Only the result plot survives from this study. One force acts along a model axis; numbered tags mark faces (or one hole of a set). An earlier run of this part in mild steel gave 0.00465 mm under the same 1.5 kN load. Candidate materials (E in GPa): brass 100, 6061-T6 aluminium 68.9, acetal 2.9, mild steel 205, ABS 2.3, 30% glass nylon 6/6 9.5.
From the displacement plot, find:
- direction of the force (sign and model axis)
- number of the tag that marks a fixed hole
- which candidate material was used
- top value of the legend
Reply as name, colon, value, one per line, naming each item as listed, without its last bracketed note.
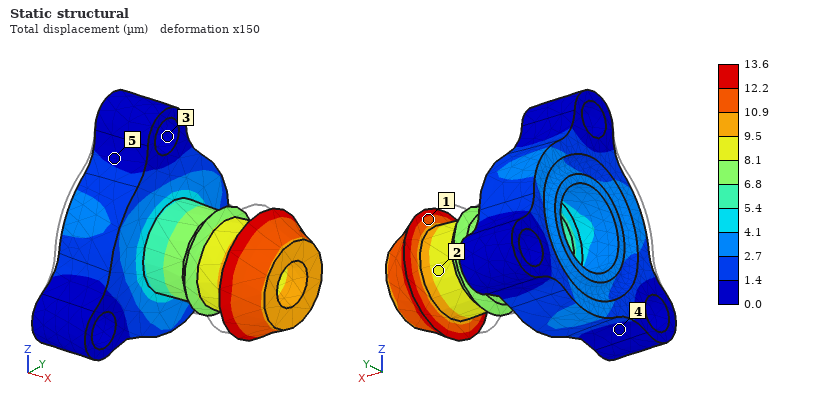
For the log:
direction of the force: +X
number of the tag that marks a fixed hole: 3
which candidate material was used: 6061-T6 aluminium
top value of the legend: 13.6 µm
